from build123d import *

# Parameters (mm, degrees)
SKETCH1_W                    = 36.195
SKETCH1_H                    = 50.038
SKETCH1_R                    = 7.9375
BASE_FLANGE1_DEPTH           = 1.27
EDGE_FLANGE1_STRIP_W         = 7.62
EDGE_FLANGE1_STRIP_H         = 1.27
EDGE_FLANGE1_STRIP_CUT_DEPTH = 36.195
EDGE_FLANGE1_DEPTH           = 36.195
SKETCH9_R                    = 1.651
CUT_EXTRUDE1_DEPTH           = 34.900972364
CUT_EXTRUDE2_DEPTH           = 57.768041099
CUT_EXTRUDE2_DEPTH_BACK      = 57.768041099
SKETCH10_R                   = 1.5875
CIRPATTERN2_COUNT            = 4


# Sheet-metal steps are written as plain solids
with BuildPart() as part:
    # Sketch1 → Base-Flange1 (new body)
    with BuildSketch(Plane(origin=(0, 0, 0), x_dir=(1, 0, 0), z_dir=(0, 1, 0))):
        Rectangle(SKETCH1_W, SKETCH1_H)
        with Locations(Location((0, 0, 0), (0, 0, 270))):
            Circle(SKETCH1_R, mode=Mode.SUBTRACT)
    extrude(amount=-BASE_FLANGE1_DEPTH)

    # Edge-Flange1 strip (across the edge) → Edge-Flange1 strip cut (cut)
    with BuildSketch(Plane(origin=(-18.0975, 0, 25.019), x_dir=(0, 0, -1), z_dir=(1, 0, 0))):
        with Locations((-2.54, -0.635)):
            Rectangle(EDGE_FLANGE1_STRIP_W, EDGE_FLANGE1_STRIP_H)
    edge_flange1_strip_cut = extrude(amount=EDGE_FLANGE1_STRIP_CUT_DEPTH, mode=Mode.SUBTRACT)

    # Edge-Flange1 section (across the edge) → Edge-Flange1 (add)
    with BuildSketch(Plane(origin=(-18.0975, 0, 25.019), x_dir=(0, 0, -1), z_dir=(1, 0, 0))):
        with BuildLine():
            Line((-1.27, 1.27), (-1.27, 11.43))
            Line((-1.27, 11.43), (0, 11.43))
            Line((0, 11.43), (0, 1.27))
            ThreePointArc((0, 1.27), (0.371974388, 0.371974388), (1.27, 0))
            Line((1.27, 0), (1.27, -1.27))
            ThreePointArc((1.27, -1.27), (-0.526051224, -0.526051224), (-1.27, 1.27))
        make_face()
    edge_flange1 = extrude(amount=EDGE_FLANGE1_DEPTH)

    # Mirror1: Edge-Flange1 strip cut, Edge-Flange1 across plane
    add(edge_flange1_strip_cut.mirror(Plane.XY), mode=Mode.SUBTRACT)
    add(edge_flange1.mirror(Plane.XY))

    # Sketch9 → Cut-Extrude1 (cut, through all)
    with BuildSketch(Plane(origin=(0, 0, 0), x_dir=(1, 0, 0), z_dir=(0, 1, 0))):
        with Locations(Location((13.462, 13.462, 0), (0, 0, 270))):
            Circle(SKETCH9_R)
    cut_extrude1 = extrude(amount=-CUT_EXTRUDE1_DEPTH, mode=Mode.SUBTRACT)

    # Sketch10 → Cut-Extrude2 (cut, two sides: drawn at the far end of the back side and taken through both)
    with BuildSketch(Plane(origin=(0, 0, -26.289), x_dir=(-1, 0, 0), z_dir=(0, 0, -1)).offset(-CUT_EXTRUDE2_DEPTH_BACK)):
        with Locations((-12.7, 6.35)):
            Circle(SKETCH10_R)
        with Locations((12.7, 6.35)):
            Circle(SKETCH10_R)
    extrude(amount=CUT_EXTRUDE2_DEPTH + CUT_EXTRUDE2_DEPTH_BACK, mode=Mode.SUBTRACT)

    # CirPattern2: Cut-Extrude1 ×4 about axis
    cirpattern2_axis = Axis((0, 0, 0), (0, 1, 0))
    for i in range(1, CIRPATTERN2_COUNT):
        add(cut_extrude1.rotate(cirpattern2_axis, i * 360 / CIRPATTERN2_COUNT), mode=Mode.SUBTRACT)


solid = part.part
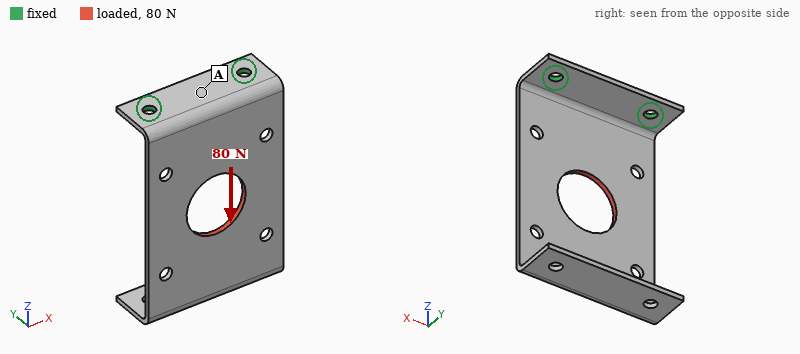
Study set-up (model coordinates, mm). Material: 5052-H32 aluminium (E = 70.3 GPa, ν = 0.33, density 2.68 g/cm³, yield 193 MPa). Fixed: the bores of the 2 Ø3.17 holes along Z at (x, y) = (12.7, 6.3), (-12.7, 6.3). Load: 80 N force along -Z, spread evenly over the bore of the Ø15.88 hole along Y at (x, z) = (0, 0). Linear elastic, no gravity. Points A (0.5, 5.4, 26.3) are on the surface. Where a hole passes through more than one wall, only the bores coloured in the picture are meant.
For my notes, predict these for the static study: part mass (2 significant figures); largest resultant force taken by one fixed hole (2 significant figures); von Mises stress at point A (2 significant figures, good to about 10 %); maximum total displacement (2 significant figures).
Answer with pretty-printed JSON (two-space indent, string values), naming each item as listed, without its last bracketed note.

{
  "part mass": "8.2 g",
  "largest resultant force taken by one fixed hole": "40 N",
  "von Mises stress at point A": "8.7 MPa",
  "maximum total displacement": "0.22 mm"
}
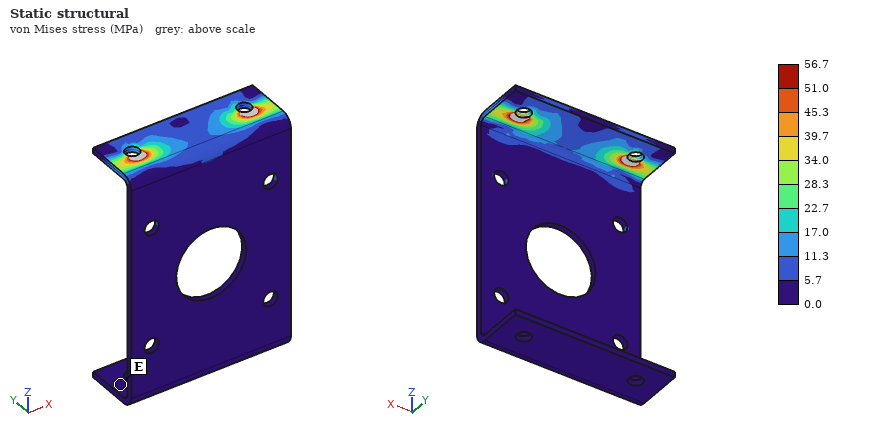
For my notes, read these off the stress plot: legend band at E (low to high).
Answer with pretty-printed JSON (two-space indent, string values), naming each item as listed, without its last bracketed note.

{
  "legend band at E": "0.0 to 5.7 MPa"
}
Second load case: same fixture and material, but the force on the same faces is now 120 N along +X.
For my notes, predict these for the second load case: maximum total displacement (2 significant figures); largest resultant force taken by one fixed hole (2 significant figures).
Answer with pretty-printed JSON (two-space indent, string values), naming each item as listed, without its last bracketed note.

{
  "maximum total displacement": "0.29 mm",
  "largest resultant force taken by one fixed hole": "130 N"
}
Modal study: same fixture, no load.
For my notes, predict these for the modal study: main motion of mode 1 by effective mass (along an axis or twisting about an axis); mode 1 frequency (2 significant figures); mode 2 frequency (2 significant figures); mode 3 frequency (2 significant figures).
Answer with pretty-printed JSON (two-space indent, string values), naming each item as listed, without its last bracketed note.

{
  "main motion of mode 1 by effective mass": "along Y",
  "mode 1 frequency": "240 Hz",
  "mode 2 frequency": "800 Hz",
  "mode 3 frequency": "1500 Hz"
}
